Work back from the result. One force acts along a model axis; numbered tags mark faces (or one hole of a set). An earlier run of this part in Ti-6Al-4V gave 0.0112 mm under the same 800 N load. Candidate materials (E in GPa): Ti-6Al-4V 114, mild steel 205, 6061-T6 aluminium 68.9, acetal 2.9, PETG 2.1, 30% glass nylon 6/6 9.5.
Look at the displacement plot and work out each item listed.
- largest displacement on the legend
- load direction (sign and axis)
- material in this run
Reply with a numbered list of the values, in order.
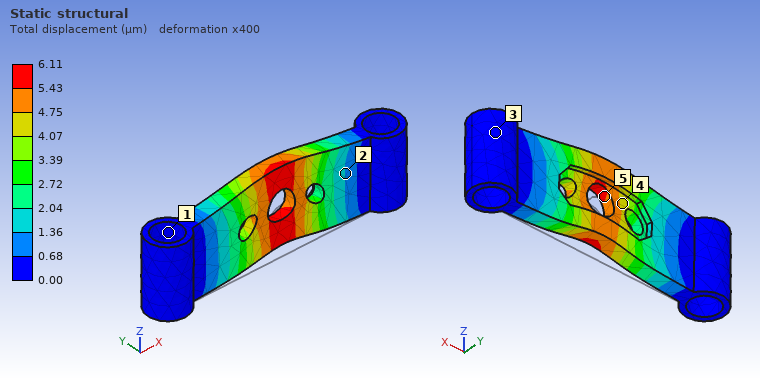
1. 6.11 µm
2. +Z
3. mild steel
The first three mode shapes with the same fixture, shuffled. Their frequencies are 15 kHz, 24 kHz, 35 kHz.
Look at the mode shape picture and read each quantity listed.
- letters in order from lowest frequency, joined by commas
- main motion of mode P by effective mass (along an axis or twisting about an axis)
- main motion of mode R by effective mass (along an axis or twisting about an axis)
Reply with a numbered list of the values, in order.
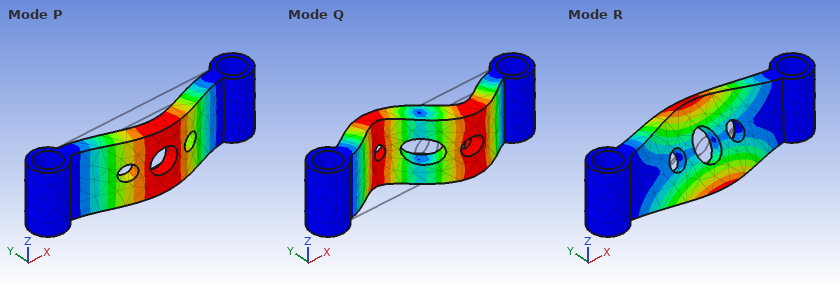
1. P, R, Q
2. along Y
3. twisting about X
